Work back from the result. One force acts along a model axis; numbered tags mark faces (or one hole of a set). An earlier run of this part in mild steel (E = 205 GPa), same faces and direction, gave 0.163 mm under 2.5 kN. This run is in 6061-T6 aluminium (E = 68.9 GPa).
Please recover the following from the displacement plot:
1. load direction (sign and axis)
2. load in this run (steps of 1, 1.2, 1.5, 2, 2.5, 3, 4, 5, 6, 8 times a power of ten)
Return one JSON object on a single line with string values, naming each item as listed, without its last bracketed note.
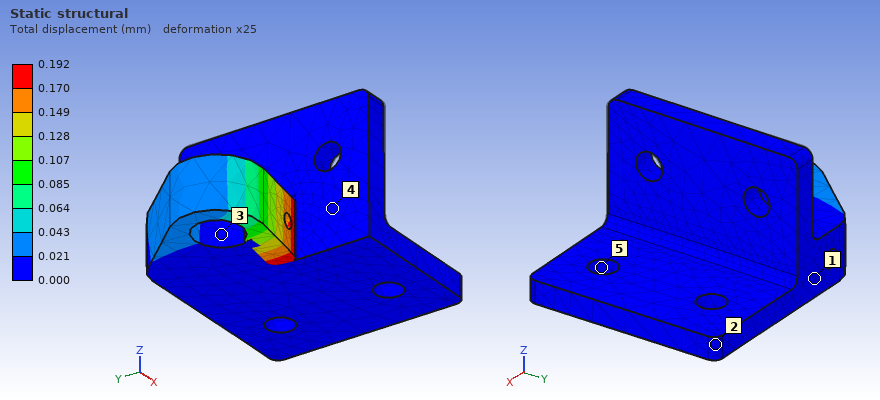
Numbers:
{"load direction": "+Y", "load in this run": "1 kN"}
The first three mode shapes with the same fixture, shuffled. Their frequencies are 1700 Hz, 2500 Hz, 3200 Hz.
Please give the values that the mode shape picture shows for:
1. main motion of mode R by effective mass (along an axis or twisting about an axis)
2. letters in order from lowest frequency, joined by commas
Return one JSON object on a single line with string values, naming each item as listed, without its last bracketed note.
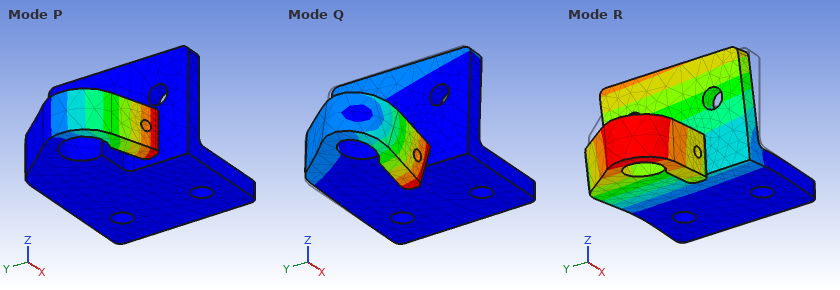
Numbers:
{"main motion of mode R by effective mass": "along Z", "letters in order from lowest frequency, joined by commas": "R, P, Q"}
